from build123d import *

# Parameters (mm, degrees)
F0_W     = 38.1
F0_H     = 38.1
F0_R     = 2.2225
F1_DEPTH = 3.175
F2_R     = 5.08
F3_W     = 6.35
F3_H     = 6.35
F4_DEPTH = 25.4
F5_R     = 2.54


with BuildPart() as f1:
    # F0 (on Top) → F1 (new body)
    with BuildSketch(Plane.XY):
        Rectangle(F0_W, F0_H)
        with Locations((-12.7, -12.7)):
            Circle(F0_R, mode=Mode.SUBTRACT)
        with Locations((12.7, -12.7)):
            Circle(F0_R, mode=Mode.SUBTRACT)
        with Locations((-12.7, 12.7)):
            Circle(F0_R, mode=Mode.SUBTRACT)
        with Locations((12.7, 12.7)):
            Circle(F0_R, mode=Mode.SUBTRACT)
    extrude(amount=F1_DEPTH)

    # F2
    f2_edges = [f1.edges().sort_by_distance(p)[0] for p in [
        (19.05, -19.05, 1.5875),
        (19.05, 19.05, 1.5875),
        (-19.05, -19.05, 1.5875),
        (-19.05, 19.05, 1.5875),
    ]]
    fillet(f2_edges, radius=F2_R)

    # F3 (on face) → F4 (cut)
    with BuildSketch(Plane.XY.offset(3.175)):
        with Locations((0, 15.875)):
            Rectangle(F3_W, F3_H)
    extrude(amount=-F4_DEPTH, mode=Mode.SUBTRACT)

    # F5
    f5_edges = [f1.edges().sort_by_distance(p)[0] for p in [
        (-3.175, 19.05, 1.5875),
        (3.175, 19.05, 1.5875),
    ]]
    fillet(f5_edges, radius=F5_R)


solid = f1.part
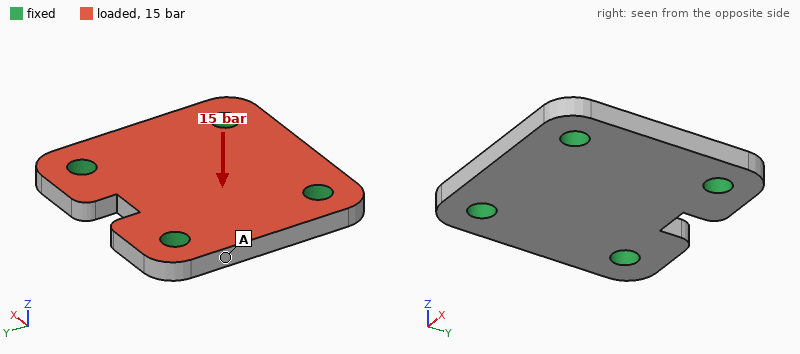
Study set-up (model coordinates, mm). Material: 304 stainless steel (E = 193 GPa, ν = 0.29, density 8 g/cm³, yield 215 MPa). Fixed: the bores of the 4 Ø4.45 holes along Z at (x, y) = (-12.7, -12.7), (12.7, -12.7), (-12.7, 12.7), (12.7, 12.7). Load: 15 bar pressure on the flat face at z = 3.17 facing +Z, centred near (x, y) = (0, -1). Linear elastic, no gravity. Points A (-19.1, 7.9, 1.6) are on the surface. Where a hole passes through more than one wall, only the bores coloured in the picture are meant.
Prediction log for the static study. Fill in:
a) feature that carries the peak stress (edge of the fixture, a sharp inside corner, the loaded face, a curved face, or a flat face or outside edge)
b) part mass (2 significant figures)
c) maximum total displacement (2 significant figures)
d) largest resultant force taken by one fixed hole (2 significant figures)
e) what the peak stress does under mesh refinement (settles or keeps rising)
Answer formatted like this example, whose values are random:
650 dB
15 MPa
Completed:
edge of the fixture
34 g
5.7 µm
510 N
keeps rising
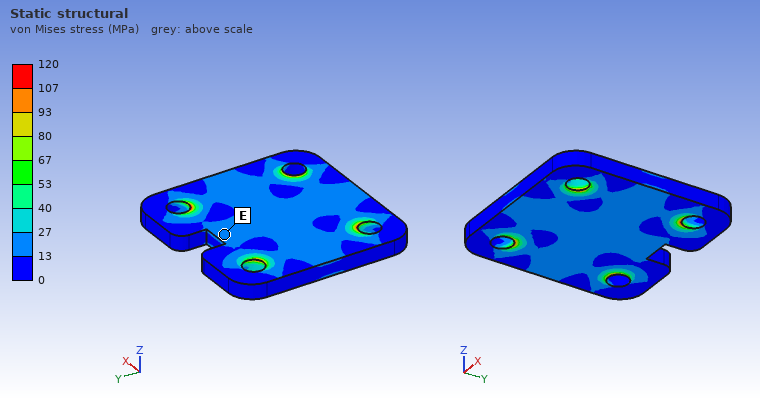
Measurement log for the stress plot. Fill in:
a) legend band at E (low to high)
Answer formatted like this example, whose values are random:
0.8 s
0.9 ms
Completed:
13 to 27 MPa
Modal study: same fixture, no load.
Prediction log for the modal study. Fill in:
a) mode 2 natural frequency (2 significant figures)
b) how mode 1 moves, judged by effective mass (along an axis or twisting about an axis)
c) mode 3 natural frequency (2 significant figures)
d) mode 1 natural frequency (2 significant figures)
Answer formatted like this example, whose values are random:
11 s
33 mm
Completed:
28 kHz
along Z
28 kHz
20 kHz
